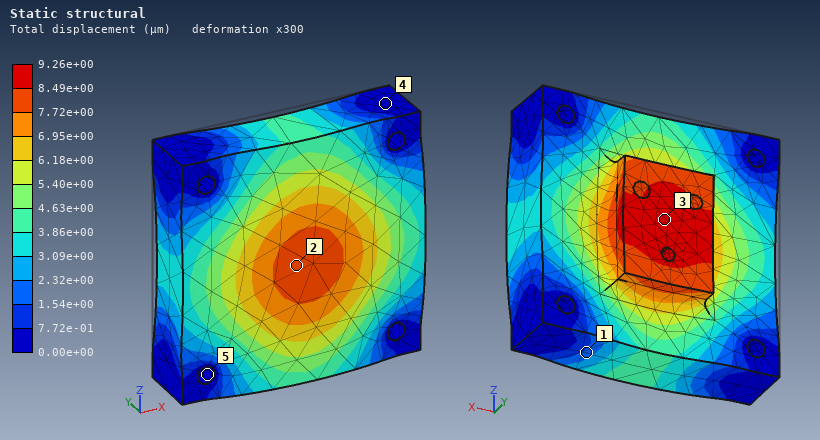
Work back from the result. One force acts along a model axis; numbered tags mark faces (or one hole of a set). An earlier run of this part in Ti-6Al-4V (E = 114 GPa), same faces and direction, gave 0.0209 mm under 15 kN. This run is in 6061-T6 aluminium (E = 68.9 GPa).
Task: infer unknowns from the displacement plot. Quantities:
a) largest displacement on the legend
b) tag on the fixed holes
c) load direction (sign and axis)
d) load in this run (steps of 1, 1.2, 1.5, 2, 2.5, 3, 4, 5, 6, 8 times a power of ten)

9.26e+00 µm
5
-Y
4 kN
